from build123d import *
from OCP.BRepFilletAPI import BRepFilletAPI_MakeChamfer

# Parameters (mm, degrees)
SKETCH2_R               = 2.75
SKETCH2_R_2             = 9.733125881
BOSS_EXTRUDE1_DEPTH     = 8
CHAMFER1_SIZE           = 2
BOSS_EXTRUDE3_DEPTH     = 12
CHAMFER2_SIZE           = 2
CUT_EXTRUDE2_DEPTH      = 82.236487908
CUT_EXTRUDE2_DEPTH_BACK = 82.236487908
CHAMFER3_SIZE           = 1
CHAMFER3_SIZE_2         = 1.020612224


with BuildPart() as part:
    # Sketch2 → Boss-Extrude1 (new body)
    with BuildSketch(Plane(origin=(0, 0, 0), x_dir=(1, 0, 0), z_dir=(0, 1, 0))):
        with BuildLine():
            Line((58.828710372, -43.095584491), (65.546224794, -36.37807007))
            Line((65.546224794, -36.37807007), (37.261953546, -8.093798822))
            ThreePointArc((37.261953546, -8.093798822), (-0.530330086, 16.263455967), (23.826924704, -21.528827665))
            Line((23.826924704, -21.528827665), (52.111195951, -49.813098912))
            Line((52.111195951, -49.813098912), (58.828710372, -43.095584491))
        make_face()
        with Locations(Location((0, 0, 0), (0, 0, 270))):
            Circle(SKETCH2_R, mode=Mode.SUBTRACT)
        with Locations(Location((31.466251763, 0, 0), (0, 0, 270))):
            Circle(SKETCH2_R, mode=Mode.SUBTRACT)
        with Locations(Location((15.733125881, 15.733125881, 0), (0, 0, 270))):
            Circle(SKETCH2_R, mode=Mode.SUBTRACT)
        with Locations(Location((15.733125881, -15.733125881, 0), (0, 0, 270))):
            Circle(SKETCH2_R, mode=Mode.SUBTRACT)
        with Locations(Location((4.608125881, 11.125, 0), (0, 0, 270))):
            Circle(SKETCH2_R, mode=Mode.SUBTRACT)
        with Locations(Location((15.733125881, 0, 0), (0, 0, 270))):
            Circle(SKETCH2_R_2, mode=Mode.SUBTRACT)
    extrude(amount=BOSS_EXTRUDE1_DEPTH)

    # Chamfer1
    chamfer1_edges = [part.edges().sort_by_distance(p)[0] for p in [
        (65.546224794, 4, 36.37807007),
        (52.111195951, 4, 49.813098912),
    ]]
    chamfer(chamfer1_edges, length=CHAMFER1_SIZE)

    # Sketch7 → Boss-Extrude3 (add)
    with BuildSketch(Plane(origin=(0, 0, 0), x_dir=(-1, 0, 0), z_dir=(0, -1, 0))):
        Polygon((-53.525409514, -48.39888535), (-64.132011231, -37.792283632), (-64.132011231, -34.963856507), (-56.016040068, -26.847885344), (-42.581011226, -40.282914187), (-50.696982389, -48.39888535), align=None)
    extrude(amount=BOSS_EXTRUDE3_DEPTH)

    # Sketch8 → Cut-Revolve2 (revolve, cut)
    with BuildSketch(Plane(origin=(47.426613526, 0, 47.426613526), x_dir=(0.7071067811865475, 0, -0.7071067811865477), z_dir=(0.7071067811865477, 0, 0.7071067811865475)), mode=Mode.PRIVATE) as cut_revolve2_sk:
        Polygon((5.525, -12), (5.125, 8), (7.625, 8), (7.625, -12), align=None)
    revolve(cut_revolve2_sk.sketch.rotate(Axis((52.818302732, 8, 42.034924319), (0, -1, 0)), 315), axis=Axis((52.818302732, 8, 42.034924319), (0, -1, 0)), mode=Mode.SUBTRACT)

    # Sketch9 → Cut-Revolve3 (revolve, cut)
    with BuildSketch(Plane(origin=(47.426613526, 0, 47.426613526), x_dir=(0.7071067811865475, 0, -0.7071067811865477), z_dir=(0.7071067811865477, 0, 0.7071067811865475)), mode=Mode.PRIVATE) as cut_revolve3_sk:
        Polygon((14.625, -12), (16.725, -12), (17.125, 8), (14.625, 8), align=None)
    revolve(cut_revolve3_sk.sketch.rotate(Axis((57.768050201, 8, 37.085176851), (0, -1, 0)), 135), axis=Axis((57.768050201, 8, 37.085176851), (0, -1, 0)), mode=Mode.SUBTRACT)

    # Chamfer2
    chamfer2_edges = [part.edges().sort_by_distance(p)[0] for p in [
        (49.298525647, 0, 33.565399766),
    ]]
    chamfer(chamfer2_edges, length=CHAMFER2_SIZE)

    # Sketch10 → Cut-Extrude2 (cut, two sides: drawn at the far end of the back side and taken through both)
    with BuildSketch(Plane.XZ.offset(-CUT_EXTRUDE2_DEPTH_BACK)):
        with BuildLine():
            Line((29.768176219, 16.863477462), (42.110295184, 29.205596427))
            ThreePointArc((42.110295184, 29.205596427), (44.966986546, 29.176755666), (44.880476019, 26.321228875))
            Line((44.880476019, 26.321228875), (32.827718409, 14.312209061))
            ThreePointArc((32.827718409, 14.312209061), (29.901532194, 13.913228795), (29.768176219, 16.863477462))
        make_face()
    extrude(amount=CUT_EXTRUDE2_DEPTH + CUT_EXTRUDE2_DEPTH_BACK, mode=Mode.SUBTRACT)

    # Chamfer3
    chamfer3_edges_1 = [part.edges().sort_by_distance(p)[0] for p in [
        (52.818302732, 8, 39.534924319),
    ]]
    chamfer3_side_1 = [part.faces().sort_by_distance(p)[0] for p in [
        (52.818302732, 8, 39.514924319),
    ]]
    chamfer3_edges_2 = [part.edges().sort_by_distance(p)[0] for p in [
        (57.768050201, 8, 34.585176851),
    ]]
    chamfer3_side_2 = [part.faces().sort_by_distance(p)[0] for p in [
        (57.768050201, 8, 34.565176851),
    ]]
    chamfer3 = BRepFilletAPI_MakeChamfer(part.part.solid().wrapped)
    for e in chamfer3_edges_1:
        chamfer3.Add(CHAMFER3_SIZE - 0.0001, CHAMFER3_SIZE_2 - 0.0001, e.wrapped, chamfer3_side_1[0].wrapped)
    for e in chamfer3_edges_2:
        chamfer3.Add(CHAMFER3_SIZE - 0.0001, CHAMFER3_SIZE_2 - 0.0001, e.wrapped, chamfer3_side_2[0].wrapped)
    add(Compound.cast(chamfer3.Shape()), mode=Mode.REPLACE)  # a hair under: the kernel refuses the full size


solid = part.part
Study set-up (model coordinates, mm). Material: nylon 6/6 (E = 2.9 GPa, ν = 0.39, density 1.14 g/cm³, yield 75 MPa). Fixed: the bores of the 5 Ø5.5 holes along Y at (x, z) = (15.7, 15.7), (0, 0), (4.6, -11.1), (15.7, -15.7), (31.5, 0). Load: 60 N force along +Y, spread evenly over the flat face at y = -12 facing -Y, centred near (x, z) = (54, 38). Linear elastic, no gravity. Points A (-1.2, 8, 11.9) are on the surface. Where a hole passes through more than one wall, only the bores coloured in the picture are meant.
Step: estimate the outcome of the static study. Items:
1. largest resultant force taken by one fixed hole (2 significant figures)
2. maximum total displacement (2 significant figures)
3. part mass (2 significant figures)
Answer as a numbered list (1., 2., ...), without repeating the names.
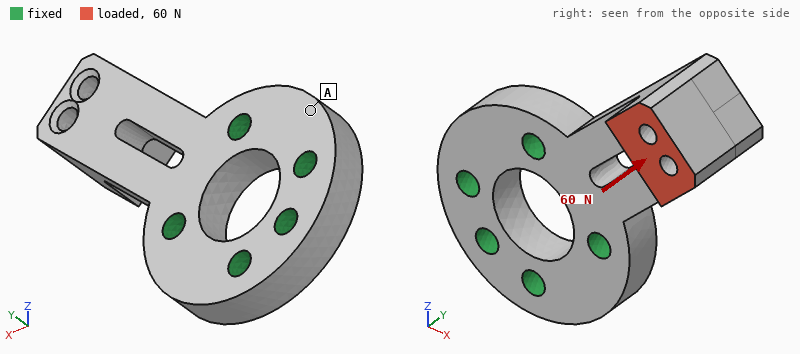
1. 33 N
2. 0.96 mm
3. 20 g
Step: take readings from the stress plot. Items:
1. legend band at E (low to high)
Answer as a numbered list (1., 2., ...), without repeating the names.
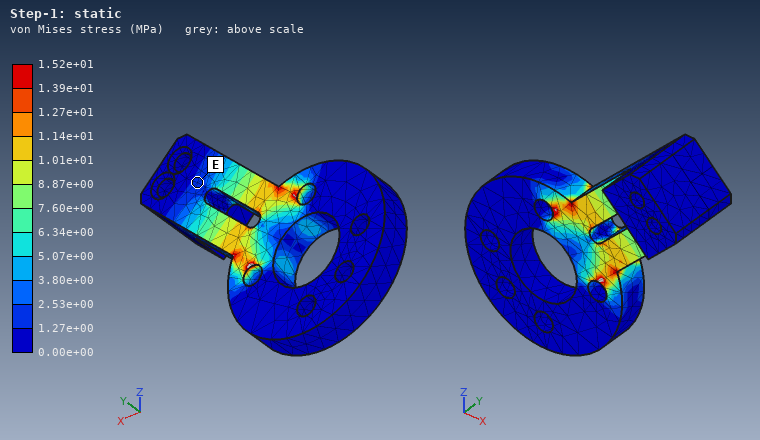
1. 1.27e+00 to 2.53e+00 MPa
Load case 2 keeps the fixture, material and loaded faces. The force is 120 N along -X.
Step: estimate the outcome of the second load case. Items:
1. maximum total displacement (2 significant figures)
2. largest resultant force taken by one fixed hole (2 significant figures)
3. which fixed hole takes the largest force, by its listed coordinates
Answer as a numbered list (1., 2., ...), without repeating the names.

1. 1.2 mm
2. 210 N
3. (15.7, 15.7)
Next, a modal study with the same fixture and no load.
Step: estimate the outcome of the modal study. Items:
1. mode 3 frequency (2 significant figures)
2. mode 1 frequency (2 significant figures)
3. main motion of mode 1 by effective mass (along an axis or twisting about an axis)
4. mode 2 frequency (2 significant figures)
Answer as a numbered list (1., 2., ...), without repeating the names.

1. 2100 Hz
2. 590 Hz
3. along Y
4. 1200 Hz
